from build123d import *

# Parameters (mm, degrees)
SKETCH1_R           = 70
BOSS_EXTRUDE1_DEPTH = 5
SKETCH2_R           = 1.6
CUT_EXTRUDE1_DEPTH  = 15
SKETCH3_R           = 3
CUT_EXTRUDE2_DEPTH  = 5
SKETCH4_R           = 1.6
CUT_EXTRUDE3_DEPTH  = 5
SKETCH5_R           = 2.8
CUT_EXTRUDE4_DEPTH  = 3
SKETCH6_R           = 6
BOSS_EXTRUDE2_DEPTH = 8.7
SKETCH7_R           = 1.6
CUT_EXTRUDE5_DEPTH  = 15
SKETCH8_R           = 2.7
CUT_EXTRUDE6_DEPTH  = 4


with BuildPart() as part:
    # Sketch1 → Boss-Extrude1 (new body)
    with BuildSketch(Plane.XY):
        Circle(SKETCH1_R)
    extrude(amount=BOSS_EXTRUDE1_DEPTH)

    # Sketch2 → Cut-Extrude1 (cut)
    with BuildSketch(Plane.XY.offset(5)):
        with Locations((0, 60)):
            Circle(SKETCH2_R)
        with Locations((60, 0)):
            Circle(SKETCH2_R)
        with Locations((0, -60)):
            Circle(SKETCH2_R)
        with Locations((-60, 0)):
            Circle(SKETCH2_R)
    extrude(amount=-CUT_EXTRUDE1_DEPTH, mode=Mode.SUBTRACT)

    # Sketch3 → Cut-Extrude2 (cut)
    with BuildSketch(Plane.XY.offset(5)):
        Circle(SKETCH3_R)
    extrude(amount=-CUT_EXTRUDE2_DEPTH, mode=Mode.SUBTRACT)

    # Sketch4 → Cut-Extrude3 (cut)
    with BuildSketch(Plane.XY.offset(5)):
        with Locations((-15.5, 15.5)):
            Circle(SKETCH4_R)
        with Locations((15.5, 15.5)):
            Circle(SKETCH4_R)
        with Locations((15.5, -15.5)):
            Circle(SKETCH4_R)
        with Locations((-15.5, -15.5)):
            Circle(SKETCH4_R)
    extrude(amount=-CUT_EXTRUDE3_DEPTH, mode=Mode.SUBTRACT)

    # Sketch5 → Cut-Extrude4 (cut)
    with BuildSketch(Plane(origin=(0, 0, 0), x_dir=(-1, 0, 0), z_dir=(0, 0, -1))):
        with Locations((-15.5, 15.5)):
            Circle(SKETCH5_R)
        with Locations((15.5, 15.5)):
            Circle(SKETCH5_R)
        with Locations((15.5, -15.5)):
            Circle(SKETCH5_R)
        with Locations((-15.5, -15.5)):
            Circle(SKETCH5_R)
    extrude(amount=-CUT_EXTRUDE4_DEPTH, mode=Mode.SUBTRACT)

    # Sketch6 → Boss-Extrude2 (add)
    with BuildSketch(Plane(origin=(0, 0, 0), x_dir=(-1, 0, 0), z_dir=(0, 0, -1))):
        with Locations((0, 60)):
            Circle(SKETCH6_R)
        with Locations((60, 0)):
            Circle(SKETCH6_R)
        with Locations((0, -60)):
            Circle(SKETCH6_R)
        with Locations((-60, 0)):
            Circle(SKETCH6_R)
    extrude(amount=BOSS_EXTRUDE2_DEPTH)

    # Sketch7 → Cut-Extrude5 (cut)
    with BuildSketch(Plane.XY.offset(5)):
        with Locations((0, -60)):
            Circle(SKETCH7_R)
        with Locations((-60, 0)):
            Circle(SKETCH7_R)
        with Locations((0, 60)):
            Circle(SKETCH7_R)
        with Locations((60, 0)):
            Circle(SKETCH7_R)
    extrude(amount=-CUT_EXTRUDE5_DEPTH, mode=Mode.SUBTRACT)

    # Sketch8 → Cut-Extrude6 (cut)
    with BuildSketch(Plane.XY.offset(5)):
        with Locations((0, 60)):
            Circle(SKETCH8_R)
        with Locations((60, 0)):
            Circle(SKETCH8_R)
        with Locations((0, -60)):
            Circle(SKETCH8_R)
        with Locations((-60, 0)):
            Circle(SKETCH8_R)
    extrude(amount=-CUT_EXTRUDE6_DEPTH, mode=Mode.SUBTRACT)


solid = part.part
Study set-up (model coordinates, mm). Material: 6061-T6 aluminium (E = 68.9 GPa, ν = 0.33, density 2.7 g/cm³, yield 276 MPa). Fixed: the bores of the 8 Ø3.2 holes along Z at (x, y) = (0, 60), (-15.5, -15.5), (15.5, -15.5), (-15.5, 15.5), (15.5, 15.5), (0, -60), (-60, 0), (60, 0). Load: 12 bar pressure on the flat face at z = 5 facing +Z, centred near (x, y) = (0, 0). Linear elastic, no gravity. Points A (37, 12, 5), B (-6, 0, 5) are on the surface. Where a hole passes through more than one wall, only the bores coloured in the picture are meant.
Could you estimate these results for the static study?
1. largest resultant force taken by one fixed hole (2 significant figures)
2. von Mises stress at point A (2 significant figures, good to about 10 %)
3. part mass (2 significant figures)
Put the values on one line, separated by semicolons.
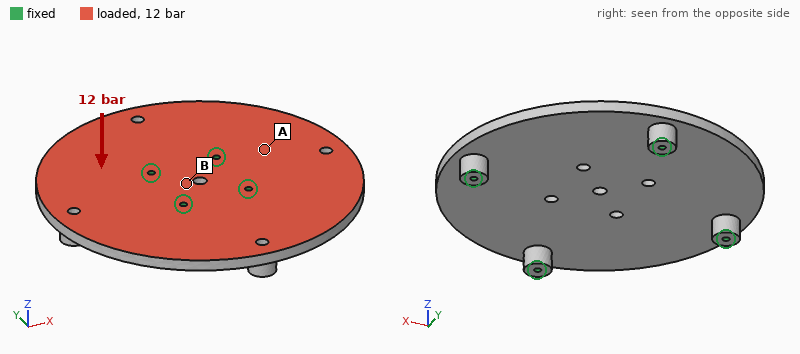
3.1 kN; 63 MPa; 220 g
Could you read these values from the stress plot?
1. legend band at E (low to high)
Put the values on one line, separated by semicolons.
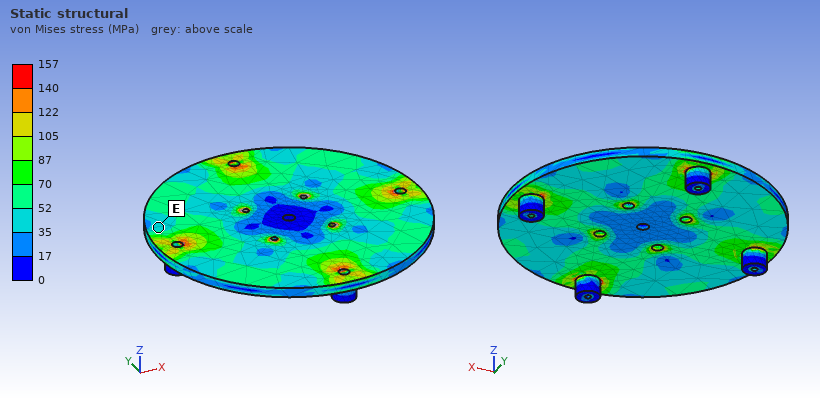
35 to 52 MPa
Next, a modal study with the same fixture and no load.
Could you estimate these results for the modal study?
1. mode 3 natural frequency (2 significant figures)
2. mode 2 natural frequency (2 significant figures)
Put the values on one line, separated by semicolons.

3300 Hz; 3300 Hz
